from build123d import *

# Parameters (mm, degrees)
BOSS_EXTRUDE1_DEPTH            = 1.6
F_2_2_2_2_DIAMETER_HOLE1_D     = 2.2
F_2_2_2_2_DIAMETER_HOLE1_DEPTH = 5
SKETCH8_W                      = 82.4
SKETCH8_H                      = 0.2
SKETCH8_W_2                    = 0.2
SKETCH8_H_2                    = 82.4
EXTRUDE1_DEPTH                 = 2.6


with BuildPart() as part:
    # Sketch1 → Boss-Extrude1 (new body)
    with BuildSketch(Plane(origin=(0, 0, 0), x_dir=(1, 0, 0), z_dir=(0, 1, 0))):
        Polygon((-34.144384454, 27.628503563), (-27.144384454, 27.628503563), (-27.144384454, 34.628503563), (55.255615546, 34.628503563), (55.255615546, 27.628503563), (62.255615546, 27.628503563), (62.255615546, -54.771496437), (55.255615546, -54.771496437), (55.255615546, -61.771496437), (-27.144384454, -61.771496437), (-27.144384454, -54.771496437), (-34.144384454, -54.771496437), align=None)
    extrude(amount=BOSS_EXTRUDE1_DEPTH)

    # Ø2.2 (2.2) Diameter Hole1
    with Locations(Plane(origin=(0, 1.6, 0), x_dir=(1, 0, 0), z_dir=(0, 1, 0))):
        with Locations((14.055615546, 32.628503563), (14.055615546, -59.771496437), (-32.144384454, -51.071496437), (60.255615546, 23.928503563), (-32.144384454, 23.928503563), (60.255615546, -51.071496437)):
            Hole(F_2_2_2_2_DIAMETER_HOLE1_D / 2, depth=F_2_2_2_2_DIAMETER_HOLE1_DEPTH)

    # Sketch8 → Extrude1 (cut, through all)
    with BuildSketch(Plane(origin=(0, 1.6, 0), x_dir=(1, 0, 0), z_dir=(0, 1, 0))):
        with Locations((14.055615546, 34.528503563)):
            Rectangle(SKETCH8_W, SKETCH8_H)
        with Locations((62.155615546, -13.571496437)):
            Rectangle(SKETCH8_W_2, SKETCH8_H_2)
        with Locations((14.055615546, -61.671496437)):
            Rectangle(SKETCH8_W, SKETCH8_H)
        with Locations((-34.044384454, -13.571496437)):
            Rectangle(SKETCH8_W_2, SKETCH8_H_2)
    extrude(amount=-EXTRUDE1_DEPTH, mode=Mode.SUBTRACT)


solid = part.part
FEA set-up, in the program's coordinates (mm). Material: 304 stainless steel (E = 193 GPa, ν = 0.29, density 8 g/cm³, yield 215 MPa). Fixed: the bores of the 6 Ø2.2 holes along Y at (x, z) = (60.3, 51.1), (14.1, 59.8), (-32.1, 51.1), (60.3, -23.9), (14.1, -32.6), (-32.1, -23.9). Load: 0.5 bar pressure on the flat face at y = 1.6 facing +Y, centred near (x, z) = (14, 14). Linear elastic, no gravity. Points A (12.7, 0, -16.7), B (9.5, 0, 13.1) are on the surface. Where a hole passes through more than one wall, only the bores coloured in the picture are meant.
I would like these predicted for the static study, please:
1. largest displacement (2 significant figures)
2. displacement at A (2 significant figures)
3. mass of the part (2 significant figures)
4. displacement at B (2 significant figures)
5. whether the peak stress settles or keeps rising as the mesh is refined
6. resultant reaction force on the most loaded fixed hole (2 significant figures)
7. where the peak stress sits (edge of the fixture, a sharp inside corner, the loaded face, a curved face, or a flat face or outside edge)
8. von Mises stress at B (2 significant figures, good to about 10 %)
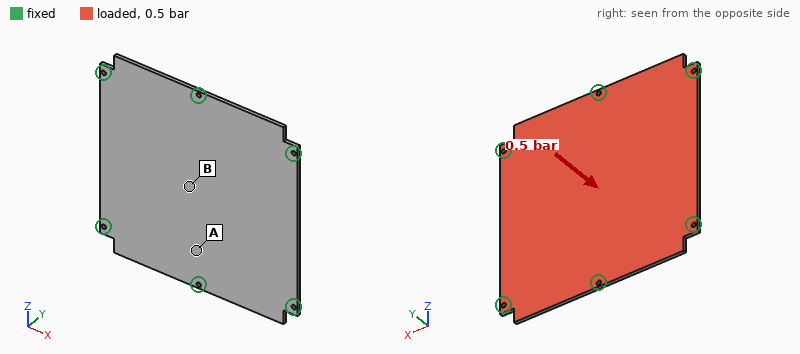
0.17 mm
0.071 mm
120 g
0.17 mm
keeps rising
98 N
edge of the fixture
40 MPa
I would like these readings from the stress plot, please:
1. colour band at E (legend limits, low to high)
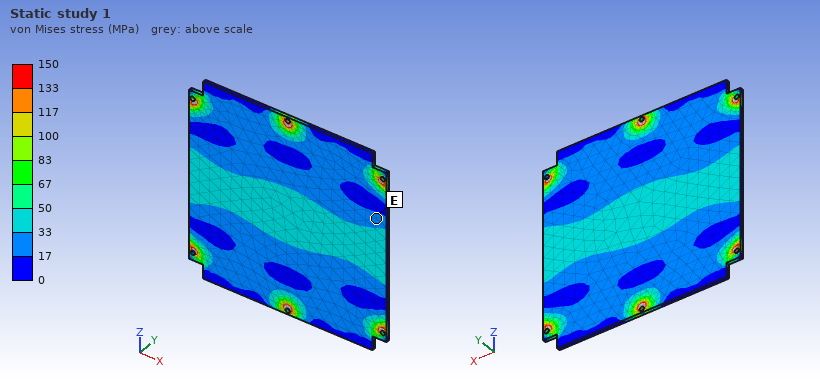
17 to 33 MPa
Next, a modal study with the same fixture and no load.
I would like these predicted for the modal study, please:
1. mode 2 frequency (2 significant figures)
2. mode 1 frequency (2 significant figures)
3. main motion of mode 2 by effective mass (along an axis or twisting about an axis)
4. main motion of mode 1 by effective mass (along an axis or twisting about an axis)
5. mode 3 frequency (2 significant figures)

1400 Hz
910 Hz
twisting about Z
along Y
2100 Hz
